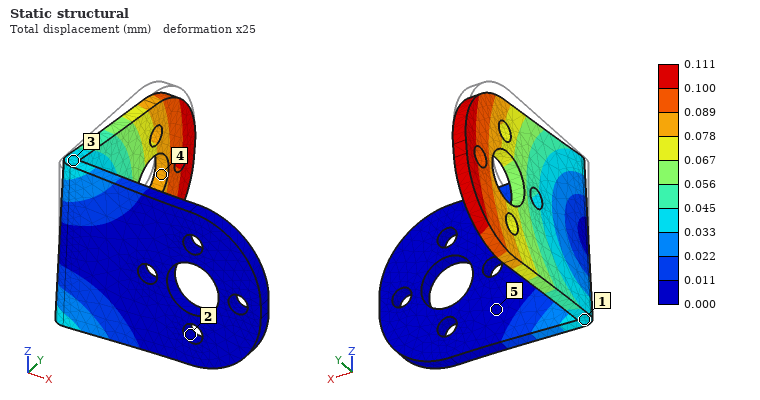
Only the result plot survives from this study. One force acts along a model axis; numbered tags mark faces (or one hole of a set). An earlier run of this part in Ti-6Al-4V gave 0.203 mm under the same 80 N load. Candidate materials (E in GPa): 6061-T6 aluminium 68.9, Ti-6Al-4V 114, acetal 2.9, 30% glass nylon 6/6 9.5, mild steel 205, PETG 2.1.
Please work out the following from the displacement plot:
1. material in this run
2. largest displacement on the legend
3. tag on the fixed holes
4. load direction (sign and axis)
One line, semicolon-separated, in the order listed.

mild steel; 0.111 mm; 2; -Z
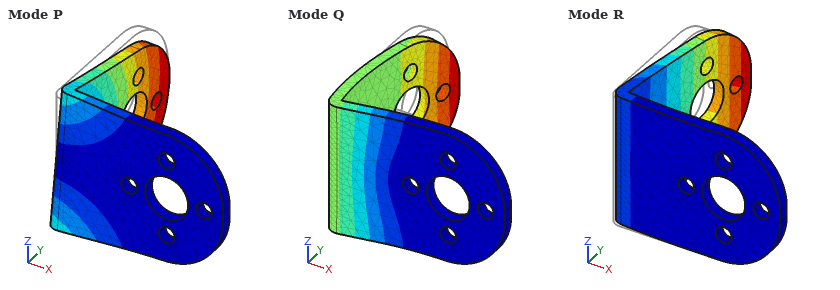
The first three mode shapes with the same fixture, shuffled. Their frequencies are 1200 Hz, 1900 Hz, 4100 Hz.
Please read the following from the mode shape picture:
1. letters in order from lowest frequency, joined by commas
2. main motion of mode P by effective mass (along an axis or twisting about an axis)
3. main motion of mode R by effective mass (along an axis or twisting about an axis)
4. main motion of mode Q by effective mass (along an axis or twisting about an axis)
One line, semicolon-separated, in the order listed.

R, P, Q; along Z; along X; along Y
